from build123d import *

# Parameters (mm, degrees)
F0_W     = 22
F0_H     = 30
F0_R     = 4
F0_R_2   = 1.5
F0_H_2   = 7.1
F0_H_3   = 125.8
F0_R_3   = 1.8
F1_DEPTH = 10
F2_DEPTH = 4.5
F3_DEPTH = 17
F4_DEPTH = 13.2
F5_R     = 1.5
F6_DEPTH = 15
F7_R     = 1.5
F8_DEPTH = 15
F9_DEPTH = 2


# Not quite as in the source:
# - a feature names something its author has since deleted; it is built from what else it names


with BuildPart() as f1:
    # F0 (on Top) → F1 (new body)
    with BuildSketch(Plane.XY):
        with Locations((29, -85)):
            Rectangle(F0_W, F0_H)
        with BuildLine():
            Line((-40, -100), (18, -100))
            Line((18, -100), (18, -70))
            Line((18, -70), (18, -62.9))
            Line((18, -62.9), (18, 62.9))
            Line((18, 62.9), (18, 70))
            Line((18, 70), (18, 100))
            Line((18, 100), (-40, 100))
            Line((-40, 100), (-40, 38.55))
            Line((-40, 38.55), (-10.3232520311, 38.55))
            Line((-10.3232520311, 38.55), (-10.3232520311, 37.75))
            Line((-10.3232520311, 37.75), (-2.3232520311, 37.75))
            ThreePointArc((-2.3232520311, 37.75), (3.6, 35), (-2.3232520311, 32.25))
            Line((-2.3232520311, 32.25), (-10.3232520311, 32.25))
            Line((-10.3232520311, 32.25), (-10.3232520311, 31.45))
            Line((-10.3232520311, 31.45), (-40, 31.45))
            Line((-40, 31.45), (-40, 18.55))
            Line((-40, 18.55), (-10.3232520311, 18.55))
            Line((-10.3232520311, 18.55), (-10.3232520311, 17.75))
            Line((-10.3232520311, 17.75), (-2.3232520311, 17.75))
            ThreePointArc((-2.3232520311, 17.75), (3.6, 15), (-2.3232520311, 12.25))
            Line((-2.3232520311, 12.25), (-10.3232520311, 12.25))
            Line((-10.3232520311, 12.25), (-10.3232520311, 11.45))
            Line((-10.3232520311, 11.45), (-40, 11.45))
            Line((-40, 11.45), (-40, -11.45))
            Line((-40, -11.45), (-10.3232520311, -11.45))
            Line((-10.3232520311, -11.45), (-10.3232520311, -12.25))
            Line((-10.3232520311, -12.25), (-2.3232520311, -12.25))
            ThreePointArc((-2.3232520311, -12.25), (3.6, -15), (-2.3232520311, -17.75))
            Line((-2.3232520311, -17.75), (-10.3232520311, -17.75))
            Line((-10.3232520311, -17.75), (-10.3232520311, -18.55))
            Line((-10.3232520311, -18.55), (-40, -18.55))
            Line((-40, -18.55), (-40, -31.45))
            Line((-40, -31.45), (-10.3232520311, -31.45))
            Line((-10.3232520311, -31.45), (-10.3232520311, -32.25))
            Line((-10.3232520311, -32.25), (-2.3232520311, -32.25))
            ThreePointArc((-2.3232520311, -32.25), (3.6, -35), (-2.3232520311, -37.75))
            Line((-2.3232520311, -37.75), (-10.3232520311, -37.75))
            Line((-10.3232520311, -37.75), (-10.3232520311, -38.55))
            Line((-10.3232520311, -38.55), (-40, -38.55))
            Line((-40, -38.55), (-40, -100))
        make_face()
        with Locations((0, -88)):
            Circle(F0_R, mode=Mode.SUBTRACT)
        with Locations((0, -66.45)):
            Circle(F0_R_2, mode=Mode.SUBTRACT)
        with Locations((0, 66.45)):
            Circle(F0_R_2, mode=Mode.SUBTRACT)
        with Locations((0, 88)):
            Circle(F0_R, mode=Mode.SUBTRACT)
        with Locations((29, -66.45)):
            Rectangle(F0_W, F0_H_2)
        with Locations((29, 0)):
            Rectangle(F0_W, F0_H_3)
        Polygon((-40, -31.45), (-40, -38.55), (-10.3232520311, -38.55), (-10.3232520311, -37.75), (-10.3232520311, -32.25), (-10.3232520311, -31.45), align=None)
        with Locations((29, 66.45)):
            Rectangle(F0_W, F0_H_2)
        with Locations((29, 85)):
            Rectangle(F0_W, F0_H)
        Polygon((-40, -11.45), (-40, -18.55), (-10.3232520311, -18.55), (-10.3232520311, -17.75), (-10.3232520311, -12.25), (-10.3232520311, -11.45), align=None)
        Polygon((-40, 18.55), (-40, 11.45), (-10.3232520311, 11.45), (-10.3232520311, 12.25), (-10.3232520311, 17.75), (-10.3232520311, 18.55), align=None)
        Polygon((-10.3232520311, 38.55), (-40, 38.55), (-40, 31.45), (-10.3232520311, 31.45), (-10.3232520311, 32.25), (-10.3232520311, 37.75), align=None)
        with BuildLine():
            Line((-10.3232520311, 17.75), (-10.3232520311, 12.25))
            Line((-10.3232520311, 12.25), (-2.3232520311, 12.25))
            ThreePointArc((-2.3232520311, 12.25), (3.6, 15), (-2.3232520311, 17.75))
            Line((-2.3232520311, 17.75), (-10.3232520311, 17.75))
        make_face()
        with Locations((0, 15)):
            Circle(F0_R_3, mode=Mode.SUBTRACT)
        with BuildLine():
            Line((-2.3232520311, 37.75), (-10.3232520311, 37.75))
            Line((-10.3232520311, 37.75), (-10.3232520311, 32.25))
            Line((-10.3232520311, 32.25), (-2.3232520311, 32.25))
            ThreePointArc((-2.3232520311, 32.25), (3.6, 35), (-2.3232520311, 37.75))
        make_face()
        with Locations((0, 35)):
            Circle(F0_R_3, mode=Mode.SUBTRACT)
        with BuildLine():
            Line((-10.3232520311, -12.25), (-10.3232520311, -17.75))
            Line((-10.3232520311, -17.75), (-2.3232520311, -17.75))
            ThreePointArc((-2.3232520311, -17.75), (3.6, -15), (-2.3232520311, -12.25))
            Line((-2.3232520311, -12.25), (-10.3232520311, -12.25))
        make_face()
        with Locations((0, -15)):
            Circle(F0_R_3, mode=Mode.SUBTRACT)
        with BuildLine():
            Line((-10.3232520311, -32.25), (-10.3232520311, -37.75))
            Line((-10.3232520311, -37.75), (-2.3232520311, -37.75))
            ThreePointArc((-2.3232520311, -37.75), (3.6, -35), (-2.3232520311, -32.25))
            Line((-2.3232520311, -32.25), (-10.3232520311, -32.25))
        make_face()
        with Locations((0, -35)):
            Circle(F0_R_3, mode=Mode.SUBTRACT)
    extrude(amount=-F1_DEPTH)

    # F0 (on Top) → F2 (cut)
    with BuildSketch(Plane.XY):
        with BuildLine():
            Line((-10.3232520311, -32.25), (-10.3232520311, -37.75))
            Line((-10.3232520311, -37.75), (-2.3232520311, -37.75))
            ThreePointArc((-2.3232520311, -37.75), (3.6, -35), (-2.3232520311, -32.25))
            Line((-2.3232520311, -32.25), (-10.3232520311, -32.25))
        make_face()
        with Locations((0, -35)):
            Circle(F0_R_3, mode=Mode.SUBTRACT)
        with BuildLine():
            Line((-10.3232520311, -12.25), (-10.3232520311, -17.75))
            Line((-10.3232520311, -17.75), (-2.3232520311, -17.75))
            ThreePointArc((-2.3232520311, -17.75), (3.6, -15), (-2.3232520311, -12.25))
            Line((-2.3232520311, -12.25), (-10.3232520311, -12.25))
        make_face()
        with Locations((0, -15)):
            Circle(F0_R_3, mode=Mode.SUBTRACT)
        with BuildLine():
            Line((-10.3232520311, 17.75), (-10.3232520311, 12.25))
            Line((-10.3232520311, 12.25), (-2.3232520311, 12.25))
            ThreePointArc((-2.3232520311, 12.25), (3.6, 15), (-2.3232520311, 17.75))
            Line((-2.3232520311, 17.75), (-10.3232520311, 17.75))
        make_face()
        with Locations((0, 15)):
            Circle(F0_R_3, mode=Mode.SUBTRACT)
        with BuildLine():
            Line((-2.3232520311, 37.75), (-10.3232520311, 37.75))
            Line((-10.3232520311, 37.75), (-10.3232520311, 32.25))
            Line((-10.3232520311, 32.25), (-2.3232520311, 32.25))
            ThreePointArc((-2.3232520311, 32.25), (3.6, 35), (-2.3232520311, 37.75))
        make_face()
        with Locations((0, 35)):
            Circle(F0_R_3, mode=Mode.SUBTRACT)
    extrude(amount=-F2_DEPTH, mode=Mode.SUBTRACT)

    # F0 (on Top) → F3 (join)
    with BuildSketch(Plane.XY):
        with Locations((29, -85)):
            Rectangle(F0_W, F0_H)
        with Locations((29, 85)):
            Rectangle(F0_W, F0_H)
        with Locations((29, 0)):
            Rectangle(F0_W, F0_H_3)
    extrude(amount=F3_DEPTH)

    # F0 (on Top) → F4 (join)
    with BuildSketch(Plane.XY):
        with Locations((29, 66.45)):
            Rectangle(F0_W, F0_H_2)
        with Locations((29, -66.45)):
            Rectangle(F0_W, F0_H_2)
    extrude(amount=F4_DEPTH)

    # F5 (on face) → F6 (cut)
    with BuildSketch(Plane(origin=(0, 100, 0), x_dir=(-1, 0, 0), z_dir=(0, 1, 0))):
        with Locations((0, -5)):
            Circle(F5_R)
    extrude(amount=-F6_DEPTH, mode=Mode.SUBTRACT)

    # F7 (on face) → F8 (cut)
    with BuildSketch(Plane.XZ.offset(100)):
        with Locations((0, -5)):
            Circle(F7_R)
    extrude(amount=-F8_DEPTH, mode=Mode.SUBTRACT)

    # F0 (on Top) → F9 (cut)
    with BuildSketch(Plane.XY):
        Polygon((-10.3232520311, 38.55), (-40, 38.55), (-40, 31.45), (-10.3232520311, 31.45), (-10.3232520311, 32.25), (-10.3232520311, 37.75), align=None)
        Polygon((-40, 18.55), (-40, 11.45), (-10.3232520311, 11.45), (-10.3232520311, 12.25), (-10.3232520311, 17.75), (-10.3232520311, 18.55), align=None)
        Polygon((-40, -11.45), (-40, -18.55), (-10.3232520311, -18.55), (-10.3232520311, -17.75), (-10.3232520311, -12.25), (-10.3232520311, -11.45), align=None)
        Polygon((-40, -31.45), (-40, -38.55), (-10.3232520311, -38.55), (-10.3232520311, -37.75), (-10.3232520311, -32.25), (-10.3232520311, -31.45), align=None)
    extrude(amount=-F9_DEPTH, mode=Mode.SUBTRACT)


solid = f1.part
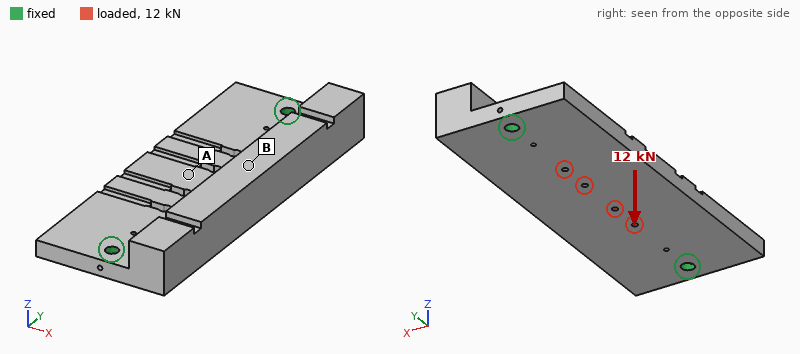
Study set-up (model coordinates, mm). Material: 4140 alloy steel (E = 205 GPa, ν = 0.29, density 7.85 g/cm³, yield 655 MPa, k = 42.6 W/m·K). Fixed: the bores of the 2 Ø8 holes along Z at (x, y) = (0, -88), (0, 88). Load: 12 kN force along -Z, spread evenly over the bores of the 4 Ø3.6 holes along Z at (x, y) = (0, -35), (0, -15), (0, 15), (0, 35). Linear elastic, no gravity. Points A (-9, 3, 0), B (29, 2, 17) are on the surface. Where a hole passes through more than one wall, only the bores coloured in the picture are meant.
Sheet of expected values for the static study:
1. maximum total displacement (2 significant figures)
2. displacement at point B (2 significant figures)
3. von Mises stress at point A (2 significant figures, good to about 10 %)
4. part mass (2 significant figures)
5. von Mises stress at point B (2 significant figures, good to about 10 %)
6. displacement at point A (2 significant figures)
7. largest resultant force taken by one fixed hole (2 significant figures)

0.17 mm
0.074 mm
33 MPa
1.8 kg
78 MPa
0.13 mm
6.8 kN
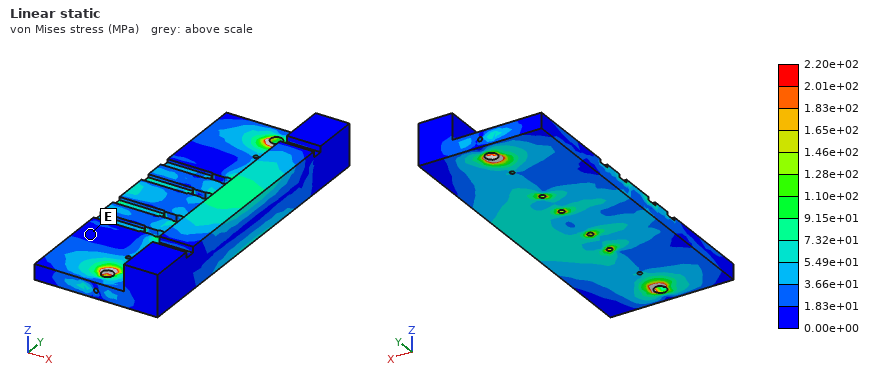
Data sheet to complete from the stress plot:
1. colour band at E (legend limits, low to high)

0.00e+00 to 1.83e+01 MPa
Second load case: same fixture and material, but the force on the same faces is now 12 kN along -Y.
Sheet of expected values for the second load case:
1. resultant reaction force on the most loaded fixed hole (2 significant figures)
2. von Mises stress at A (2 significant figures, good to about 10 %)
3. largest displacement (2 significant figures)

6.0 kN
6.8 MPa
6.3 µm
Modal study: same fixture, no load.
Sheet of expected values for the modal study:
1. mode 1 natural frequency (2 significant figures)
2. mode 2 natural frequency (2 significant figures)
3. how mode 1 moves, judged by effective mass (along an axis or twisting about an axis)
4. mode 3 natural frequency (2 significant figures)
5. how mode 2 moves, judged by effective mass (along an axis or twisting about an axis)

1500 Hz
1800 Hz
along Z
3600 Hz
along Z
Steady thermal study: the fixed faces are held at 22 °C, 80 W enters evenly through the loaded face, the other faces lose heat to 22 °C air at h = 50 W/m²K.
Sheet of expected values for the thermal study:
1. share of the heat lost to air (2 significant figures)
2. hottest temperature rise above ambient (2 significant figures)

64 %
65 K
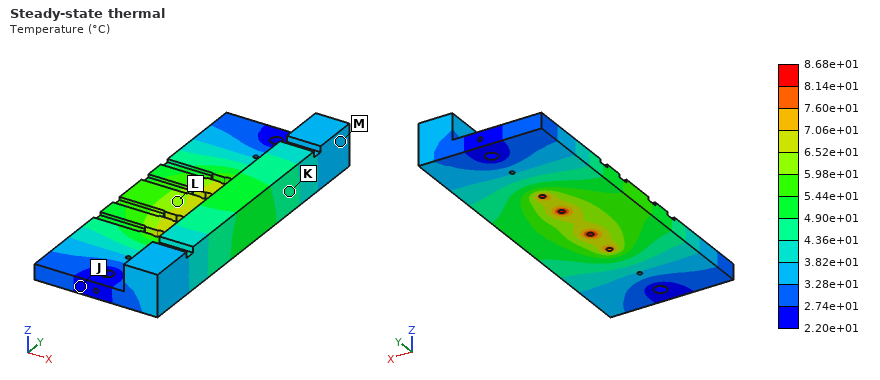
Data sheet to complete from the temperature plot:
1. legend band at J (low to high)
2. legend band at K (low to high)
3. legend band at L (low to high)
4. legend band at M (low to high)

2.20e+01 to 2.74e+01 °C
4.36e+01 to 4.90e+01 °C
5.98e+01 to 6.52e+01 °C
3.28e+01 to 3.82e+01 °C
